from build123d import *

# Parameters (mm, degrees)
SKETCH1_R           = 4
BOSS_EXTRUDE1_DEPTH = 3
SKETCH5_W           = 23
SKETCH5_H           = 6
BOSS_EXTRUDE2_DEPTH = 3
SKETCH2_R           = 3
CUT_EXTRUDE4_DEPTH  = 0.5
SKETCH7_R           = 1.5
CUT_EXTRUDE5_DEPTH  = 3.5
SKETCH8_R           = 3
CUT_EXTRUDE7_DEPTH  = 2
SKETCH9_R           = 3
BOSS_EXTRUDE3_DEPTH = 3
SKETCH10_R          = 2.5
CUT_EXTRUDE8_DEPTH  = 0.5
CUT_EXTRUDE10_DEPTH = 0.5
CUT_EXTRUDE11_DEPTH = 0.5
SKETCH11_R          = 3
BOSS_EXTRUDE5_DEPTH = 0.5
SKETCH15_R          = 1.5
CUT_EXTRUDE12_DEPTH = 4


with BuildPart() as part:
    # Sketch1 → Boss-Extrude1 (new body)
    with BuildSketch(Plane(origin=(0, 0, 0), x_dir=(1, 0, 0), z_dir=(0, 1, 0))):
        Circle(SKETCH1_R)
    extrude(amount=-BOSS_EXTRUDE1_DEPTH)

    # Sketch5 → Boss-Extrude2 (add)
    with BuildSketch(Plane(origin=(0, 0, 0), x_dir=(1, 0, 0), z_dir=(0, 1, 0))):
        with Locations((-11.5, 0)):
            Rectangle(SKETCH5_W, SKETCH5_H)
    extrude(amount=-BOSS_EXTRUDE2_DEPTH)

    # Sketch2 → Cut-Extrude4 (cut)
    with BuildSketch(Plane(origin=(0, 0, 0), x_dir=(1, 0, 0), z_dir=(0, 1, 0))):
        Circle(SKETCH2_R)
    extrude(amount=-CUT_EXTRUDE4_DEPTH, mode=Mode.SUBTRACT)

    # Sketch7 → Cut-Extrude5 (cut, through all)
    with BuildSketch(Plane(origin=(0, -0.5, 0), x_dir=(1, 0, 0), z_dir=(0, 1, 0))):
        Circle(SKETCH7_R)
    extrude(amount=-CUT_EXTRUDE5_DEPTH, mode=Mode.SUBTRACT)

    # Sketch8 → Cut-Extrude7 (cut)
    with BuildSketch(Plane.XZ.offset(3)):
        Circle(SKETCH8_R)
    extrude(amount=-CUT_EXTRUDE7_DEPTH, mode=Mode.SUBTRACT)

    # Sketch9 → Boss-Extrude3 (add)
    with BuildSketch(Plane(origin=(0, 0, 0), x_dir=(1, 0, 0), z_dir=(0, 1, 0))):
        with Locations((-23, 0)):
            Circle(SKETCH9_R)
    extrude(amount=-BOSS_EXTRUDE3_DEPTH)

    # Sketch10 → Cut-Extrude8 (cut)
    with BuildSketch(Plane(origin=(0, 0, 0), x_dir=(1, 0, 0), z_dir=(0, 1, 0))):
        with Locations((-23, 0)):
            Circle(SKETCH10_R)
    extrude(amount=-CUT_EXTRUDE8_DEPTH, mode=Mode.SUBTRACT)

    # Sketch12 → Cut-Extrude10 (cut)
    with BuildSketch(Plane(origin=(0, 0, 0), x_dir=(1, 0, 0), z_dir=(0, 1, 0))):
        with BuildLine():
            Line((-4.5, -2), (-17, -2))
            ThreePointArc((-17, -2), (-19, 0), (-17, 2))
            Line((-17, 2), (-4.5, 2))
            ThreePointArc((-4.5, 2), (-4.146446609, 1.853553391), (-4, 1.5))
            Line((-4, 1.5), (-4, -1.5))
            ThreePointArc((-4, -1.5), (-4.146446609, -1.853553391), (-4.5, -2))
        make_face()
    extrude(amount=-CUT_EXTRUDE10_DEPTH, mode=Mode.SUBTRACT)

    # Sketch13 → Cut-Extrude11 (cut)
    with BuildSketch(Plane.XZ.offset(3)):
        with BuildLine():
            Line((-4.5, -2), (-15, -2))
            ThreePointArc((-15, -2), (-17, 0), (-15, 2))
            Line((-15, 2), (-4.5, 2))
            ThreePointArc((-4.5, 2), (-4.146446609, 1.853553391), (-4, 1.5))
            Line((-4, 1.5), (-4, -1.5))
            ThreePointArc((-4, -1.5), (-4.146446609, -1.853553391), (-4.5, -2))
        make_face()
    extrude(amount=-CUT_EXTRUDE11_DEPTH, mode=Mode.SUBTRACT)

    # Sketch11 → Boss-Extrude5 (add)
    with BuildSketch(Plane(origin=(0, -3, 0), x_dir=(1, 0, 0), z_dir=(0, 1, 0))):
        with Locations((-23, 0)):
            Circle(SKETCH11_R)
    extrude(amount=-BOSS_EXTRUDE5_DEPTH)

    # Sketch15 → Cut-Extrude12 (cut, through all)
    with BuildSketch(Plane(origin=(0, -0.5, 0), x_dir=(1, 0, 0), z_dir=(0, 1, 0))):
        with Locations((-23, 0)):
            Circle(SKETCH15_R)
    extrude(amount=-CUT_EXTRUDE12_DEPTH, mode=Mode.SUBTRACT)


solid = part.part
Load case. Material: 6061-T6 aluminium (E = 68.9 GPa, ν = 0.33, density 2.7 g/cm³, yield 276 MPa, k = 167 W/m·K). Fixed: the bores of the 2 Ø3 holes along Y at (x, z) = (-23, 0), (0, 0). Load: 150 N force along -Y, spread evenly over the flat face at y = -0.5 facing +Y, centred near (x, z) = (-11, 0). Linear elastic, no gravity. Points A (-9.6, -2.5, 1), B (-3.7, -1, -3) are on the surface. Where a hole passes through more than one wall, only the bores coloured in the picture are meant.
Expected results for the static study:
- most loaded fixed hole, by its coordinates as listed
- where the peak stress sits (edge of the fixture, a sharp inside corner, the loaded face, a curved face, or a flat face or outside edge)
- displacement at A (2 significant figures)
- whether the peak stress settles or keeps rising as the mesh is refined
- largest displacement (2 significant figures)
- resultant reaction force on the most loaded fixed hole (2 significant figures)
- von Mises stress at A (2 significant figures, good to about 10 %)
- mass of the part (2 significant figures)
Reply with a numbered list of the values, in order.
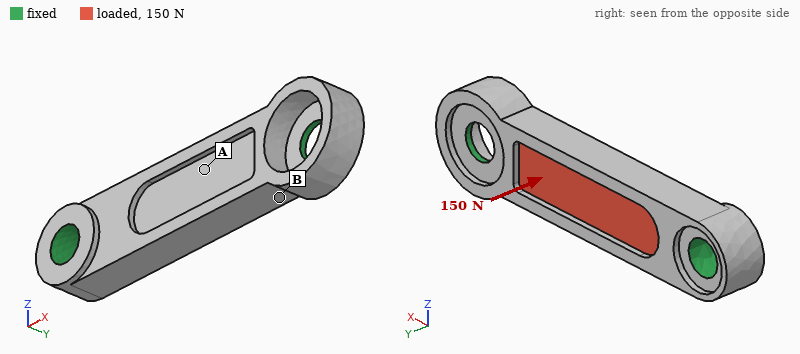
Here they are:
1. (-23, 0)
2. edge of the fixture
3. 17 µm
4. keeps rising
5. 17 µm
6. 100 N
7. 33 MPa
8. 1.1 g
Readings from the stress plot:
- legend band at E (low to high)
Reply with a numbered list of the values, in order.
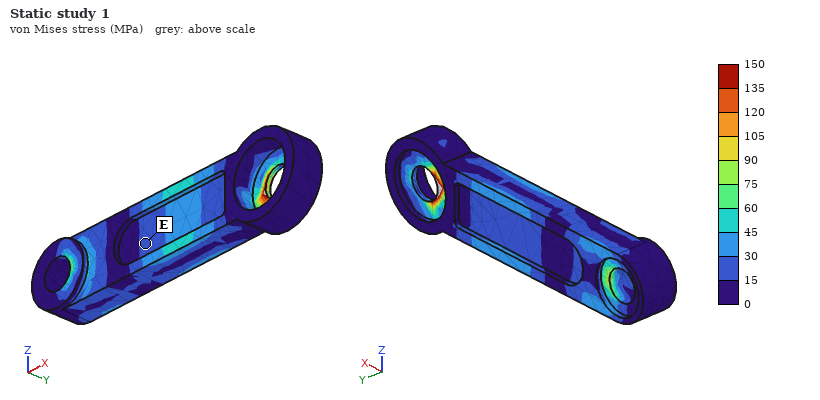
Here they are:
1. 15 to 30 MPa
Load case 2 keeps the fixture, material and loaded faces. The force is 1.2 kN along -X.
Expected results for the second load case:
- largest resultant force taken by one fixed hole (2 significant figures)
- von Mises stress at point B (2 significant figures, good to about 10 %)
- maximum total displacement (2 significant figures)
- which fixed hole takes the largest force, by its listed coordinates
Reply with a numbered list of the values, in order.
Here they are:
1. 810 N
2. 45 MPa
3. 16 µm
4. (-23, 0)
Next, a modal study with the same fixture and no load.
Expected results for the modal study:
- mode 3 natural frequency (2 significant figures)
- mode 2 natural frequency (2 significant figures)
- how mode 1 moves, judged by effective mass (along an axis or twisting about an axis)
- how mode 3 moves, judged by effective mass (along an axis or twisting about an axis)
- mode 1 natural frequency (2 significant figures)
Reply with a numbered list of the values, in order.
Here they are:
1. 39 kHz
2. 29 kHz
3. along Y
4. along Z
5. 21 kHz
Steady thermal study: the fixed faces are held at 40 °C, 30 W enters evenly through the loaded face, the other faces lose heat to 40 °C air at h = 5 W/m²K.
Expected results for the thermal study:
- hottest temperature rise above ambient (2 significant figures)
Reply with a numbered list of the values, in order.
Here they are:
1. 55 K
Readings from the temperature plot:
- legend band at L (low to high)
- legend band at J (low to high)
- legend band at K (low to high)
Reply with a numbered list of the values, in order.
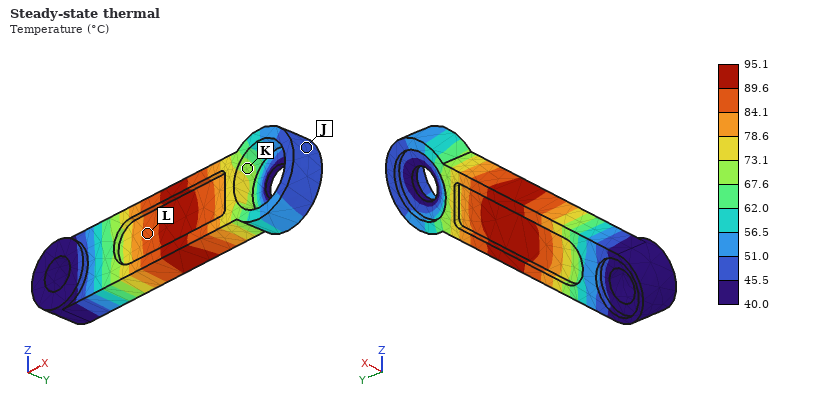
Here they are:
1. 84.1 to 89.6 °C
2. 45.5 to 51.0 °C
3. 67.6 to 73.1 °C
